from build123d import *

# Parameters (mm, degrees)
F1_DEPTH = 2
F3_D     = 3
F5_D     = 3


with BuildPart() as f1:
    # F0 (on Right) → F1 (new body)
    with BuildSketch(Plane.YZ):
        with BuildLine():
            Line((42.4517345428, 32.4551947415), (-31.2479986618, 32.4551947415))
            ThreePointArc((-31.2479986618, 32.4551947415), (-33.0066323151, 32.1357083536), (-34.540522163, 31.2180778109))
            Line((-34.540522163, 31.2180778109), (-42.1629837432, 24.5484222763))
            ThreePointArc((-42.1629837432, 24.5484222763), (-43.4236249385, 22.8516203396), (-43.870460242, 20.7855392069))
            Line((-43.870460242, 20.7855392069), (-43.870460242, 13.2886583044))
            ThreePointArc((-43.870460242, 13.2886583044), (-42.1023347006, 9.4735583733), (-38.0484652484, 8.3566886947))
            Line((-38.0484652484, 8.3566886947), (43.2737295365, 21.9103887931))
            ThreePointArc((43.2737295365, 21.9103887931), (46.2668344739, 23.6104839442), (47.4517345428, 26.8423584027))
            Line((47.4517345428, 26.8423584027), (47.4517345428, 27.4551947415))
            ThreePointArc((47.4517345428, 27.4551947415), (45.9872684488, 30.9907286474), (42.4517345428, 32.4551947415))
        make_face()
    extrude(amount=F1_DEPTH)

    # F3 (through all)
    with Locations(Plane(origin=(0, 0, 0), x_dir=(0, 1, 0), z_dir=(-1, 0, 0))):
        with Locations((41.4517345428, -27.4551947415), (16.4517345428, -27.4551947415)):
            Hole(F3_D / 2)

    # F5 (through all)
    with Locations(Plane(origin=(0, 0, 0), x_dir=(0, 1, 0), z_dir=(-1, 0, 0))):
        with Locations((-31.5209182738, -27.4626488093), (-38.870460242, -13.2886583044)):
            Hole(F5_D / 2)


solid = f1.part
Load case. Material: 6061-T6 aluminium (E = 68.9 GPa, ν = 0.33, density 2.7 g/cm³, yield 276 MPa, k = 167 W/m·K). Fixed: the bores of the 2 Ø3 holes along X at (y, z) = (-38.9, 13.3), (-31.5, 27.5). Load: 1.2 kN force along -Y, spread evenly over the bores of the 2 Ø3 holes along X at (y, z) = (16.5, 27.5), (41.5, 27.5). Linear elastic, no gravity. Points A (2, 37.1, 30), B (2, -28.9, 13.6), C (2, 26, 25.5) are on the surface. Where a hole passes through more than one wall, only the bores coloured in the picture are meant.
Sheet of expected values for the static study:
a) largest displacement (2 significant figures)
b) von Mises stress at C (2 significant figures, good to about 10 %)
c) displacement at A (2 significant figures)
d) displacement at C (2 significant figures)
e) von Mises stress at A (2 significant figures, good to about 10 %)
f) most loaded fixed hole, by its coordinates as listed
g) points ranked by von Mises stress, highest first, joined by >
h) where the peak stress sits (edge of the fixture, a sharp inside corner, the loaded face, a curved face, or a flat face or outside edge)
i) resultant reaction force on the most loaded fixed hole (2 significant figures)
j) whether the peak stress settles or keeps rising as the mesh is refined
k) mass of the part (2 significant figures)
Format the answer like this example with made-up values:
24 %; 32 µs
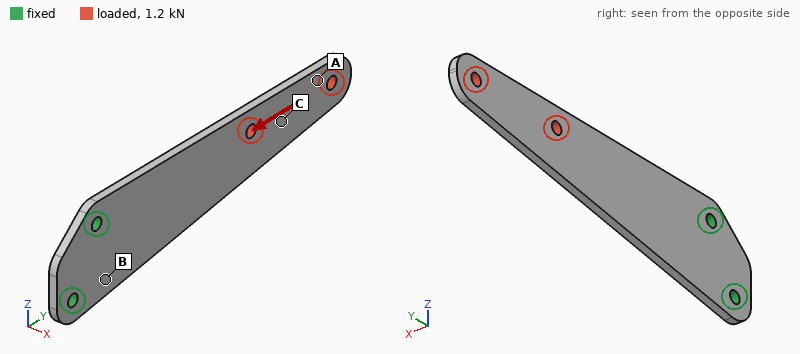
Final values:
0.21 mm; 19 MPa; 0.17 mm; 0.12 mm; 34 MPa; (-31.5, 27.5); A > C > B; edge of the fixture; 1.1 kN; keeps rising; 8.1 g
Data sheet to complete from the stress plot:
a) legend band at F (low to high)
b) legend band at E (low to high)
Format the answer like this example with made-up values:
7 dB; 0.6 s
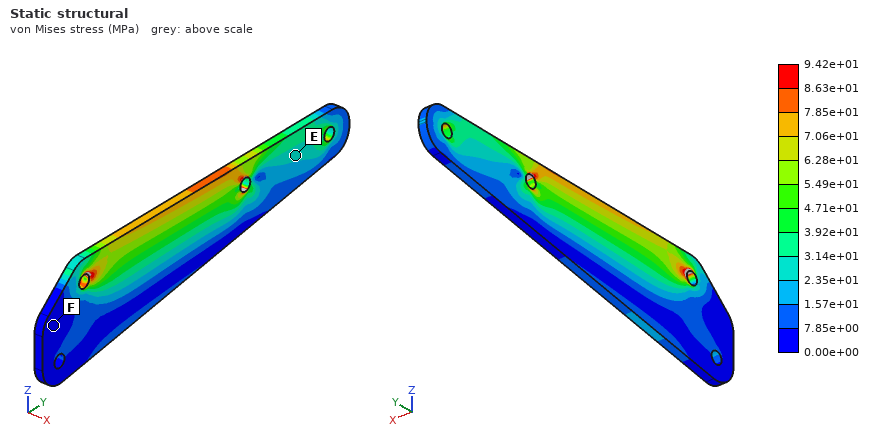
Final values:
0.00e+00 to 7.85e+00 MPa; 2.35e+01 to 3.14e+01 MPa
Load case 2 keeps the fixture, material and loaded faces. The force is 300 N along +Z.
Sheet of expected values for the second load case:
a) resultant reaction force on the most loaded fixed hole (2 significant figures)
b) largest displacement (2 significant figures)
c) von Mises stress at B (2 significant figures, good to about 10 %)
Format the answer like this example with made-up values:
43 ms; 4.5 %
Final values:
1.2 kN; 0.46 mm; 70 MPa
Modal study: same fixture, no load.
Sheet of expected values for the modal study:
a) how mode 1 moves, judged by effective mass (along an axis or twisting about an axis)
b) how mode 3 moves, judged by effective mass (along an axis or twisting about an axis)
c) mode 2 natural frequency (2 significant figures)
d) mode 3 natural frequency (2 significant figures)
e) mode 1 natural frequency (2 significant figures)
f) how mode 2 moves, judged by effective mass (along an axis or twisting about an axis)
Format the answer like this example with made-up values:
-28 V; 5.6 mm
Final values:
along X; along Z; 1800 Hz; 3100 Hz; 340 Hz; along X
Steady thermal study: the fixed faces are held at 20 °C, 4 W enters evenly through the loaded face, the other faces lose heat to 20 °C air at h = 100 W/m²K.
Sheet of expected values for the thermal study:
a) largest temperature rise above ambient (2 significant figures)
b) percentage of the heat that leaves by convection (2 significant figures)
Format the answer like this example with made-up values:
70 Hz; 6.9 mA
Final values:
22 K; 67 %
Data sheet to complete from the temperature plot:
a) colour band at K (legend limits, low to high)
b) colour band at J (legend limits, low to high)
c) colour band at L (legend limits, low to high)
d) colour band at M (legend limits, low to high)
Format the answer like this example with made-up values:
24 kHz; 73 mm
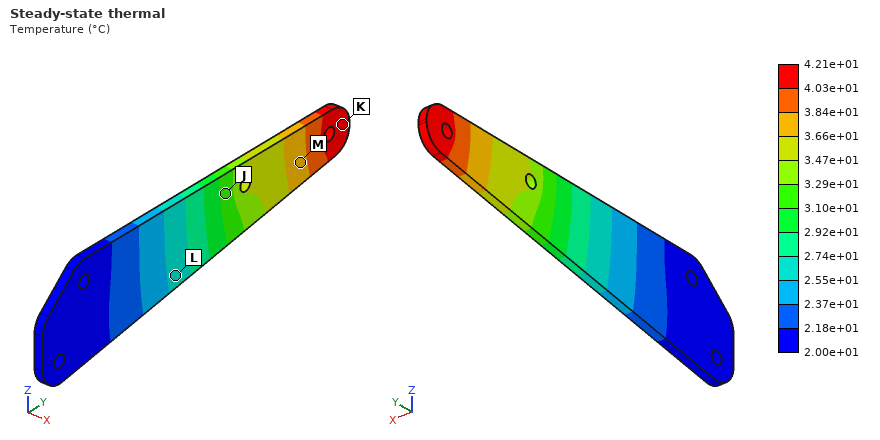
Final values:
4.03e+01 to 4.21e+01 °C; 3.10e+01 to 3.29e+01 °C; 2.55e+01 to 2.74e+01 °C; 3.66e+01 to 3.84e+01 °C
